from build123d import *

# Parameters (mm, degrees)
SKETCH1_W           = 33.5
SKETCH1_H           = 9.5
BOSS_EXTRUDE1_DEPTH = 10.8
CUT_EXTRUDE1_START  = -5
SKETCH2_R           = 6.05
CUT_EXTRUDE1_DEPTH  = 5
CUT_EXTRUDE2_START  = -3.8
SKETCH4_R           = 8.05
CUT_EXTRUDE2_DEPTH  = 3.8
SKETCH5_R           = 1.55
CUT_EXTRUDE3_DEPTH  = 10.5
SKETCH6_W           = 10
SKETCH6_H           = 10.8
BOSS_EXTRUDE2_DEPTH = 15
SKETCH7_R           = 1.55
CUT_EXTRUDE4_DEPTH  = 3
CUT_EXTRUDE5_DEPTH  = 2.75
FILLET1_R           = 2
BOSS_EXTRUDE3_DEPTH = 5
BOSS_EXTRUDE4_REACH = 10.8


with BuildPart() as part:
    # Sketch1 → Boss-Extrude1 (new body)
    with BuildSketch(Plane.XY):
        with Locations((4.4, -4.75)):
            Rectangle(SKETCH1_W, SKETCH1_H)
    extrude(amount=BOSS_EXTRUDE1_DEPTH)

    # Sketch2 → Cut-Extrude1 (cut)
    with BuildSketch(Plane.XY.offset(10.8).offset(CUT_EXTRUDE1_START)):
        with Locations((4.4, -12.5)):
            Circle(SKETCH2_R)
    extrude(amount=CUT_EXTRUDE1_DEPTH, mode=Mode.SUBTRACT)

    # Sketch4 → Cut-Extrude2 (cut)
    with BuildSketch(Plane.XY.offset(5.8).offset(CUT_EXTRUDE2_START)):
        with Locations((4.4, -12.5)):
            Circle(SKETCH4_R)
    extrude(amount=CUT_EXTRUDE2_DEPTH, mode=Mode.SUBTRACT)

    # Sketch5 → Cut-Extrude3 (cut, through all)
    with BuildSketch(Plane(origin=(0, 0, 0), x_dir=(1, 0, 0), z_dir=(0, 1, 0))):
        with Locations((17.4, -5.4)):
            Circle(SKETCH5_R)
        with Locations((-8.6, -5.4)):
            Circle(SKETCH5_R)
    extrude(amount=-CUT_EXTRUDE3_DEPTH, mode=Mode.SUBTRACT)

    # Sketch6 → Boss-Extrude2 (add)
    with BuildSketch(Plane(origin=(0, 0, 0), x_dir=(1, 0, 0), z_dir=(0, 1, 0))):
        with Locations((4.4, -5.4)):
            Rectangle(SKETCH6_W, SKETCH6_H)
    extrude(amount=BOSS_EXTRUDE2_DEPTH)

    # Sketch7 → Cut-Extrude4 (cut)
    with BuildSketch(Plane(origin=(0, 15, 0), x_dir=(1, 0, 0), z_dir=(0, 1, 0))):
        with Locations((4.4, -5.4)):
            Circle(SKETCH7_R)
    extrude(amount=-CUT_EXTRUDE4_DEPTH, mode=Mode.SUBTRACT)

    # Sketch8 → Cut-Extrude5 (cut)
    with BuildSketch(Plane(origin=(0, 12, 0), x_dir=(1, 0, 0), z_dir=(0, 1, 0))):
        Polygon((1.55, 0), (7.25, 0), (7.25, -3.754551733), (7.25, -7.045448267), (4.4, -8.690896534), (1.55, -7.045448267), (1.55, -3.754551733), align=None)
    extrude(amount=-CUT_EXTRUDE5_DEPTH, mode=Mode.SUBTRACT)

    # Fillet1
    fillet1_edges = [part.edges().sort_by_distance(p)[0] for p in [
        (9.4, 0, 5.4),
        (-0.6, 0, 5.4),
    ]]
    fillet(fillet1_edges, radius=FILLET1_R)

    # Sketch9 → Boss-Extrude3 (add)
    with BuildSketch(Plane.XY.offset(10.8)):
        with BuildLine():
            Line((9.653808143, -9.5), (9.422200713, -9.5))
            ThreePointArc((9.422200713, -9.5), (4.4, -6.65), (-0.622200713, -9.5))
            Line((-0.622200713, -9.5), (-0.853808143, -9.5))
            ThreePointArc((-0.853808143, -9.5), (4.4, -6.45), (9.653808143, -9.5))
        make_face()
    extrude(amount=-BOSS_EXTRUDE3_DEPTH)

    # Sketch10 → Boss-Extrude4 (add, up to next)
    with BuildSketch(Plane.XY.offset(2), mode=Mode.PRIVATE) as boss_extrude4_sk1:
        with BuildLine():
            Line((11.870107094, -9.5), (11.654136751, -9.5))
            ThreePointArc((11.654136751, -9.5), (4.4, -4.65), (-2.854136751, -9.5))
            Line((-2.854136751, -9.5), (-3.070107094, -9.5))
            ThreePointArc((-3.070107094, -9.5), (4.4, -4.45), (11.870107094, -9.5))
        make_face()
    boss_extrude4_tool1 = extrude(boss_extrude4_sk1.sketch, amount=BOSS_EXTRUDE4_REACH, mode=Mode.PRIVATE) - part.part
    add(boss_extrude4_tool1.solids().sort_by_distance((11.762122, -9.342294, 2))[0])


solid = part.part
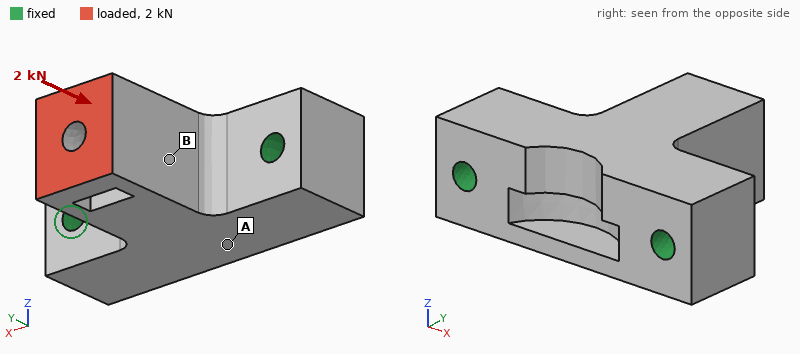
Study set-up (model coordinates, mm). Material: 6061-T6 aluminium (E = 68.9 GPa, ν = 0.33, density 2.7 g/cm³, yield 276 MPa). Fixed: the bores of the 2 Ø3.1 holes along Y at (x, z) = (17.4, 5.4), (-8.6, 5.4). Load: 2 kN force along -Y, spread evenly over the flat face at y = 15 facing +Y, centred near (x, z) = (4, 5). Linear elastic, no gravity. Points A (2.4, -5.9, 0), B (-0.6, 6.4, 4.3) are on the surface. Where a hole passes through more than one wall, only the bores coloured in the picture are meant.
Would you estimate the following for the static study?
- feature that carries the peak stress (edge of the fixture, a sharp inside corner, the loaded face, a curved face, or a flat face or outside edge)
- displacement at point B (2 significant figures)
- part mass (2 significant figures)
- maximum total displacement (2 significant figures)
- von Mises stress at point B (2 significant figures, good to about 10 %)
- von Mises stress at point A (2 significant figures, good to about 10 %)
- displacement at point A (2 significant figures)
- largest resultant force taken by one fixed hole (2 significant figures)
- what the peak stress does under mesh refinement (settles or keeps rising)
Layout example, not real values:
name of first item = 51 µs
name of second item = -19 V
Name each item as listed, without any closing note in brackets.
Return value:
feature that carries the peak stress = edge of the fixture
displacement at point B = 8.5 µm
part mass = 12 g
maximum total displacement = 18 µm
von Mises stress at point B = 31 MPa
von Mises stress at point A = 10 MPa
displacement at point A = 6.3 µm
largest resultant force taken by one fixed hole = 1.1 kN
what the peak stress does under mesh refinement = keeps rising
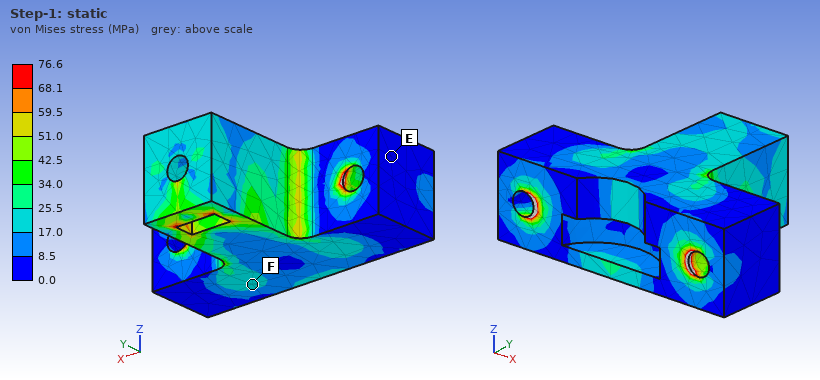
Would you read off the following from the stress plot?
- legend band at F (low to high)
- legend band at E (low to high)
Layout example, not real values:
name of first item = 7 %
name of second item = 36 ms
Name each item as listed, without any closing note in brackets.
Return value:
legend band at F = 17.0 to 25.5 MPa
legend band at E = 0.0 to 8.5 MPa
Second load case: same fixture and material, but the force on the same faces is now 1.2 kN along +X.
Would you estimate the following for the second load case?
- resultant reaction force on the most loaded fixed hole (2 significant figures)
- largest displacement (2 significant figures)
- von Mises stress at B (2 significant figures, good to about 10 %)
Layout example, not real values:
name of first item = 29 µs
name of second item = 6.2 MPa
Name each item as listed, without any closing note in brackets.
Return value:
resultant reaction force on the most loaded fixed hole = 1.3 kN
largest displacement = 61 µm
von Mises stress at B = 68 MPa
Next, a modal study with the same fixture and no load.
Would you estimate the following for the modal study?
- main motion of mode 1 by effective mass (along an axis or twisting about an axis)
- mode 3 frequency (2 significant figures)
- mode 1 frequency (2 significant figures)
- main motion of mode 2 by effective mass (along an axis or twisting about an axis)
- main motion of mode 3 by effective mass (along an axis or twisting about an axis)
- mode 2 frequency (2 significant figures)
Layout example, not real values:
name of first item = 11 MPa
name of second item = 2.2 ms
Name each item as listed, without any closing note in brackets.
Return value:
main motion of mode 1 by effective mass = along Z
mode 3 frequency = 32 kHz
mode 1 frequency = 13 kHz
main motion of mode 2 by effective mass = along X
main motion of mode 3 by effective mass = along Y
mode 2 frequency = 22 kHz
